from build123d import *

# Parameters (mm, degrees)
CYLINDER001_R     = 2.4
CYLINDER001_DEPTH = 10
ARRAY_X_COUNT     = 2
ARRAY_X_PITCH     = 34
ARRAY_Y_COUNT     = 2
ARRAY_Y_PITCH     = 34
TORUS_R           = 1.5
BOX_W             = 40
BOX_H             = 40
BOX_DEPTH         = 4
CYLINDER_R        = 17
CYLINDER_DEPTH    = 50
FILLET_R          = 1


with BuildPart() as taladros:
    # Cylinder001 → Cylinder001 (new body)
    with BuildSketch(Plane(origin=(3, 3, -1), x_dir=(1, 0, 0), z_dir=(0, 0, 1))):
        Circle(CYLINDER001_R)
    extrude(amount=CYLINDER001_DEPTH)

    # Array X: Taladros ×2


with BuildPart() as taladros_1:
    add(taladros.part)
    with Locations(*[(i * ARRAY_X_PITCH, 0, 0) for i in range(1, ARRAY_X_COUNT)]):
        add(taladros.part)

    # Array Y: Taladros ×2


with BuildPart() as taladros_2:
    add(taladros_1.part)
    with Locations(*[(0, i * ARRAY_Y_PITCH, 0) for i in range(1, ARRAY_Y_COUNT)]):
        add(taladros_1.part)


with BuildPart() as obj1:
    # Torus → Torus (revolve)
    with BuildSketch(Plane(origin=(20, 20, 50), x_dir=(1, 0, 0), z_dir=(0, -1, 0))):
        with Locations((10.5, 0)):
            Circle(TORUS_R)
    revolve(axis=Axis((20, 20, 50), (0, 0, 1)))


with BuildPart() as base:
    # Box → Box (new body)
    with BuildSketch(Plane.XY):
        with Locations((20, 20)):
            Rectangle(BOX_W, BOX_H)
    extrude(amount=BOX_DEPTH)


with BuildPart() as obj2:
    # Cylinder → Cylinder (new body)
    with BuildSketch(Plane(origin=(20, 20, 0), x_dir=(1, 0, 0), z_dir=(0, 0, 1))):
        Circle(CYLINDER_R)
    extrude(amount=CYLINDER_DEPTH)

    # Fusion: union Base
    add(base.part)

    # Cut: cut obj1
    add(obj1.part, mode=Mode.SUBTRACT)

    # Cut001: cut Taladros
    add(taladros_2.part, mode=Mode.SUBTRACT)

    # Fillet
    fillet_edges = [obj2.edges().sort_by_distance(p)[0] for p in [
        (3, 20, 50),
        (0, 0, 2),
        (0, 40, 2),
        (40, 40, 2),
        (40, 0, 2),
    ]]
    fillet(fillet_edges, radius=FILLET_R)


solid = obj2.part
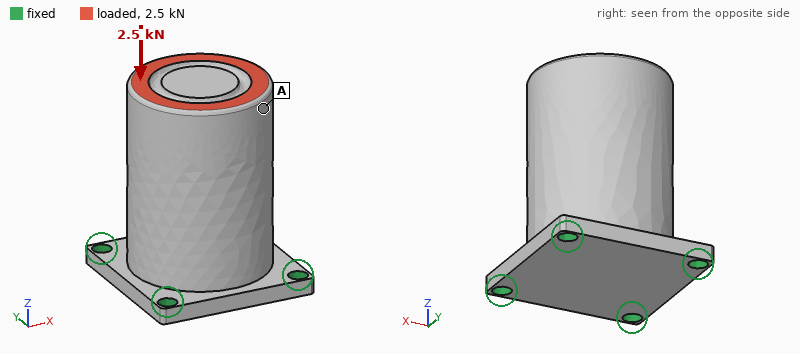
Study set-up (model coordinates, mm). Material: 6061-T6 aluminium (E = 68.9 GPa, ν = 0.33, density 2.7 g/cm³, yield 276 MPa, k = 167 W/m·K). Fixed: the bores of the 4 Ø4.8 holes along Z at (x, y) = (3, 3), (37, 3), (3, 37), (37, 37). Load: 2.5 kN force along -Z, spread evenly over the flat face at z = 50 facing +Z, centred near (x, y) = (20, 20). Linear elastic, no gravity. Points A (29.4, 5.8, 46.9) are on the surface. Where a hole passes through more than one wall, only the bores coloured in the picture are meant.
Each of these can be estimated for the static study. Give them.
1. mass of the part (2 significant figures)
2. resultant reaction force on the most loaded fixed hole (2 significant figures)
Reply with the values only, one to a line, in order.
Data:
130 g
680 N
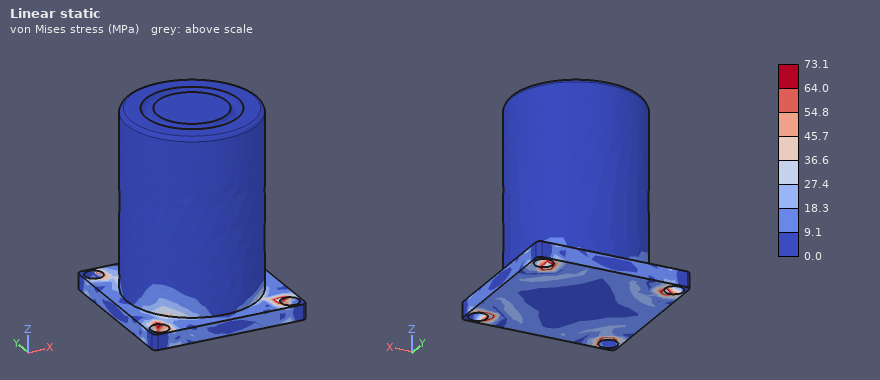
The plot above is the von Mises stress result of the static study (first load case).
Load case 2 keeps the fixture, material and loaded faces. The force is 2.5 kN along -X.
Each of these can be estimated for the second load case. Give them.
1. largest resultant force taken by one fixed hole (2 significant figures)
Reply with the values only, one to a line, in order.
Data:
2.2 kN
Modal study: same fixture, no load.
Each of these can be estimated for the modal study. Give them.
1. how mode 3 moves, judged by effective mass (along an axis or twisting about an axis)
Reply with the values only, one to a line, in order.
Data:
along Z
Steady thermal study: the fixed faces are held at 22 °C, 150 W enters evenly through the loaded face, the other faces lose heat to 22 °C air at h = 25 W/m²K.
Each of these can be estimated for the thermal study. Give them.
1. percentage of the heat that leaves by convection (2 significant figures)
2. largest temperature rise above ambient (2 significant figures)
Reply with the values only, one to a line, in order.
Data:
6.4 %
82 K
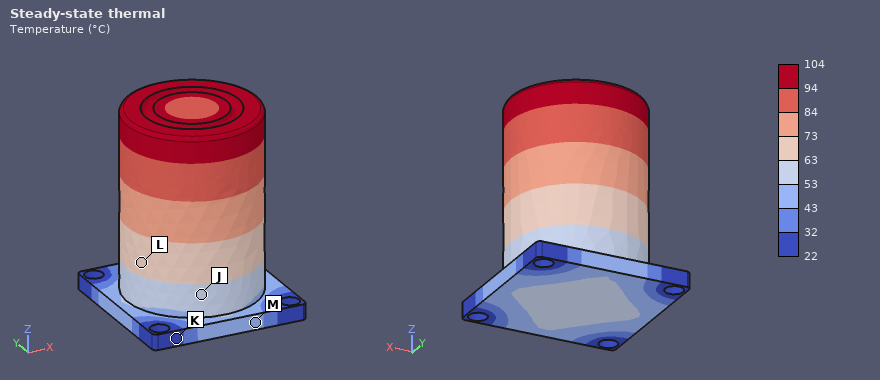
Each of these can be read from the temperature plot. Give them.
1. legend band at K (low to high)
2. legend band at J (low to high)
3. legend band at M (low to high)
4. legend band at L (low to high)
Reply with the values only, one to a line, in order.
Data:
22 to 32 °C
53 to 63 °C
43 to 53 °C
63 to 73 °C
